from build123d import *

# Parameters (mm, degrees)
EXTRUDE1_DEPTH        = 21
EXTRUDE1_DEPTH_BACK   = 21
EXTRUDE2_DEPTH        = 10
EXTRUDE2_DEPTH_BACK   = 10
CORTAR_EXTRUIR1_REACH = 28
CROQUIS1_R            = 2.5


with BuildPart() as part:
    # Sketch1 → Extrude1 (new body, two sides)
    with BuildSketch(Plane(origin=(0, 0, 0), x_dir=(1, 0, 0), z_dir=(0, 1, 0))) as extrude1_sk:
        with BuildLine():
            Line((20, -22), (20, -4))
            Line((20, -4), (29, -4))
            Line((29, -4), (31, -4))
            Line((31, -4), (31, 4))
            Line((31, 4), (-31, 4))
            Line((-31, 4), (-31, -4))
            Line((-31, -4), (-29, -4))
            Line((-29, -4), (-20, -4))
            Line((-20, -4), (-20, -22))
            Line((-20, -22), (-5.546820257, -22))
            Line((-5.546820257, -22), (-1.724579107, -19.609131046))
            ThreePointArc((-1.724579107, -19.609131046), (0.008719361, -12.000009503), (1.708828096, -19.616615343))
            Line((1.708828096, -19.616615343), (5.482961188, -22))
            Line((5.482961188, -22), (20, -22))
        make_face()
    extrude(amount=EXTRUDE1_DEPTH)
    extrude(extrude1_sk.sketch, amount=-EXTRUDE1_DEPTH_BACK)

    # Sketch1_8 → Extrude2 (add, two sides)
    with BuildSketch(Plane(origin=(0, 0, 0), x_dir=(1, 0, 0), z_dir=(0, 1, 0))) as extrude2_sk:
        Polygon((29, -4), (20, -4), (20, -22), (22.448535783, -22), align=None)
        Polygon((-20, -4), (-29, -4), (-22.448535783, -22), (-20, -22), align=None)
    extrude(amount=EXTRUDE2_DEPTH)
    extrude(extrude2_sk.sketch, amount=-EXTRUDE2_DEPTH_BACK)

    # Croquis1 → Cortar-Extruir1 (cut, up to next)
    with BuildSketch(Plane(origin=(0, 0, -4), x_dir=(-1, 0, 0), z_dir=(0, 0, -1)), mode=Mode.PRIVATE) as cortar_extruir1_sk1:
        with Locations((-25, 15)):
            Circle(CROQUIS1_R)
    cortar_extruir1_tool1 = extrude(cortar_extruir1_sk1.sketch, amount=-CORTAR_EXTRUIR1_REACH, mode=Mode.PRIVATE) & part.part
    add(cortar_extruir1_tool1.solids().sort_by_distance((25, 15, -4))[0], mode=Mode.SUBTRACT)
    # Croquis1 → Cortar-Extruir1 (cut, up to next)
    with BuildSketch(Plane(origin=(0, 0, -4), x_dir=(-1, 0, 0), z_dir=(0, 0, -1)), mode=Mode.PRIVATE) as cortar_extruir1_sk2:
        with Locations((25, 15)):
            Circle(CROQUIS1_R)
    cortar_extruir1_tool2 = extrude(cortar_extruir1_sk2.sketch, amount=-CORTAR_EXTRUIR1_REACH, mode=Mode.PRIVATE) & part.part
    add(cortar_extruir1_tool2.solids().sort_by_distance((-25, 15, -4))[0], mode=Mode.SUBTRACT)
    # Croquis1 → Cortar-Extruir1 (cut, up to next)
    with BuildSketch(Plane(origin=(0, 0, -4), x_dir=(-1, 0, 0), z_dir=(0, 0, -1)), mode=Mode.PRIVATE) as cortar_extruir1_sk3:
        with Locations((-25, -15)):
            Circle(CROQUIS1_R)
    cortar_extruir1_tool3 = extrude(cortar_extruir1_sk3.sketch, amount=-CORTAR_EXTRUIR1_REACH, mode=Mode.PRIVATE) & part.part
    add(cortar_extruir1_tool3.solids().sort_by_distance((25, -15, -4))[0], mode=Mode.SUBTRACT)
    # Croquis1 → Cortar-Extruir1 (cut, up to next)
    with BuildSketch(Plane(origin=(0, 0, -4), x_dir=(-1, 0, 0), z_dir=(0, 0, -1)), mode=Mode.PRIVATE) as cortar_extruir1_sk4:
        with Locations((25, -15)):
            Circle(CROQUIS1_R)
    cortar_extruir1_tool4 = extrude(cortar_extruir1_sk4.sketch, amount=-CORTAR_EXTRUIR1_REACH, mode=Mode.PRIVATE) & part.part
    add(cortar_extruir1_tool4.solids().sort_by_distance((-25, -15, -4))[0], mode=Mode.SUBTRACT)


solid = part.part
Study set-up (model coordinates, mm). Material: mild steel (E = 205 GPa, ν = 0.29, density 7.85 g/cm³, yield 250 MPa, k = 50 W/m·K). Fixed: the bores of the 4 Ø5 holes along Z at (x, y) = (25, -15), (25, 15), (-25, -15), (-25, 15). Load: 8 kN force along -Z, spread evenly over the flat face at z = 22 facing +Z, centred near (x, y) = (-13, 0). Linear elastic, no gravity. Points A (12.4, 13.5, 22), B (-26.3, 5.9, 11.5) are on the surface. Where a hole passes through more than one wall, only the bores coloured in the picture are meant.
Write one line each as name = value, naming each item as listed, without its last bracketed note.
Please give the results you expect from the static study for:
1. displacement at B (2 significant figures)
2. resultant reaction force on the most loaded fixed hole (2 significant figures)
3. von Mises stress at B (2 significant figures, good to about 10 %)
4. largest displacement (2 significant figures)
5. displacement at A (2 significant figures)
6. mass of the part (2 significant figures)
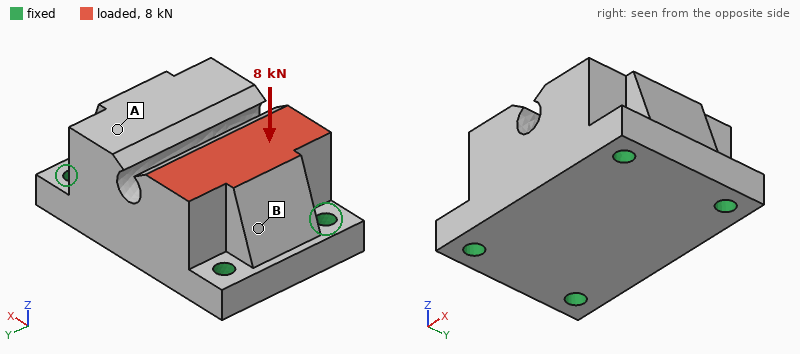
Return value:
displacement at B = 2.3 µm
resultant reaction force on the most loaded fixed hole = 3.3 kN
von Mises stress at B = 14 MPa
largest displacement = 4.0 µm
displacement at A = 2.5 µm
mass of the part = 410 g
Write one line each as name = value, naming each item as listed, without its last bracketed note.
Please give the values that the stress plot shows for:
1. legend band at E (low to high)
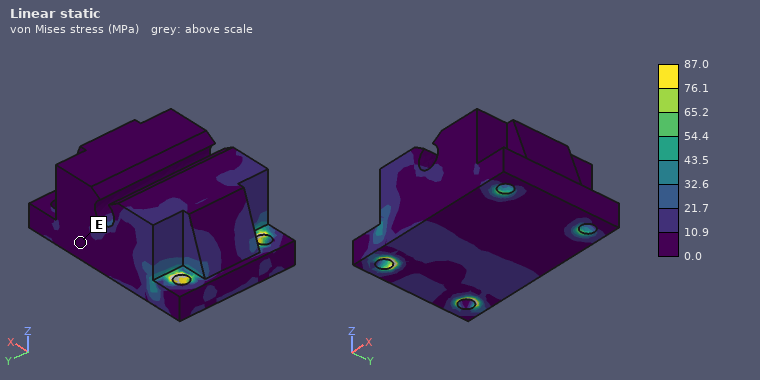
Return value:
legend band at E = 0.0 to 10.9 MPa
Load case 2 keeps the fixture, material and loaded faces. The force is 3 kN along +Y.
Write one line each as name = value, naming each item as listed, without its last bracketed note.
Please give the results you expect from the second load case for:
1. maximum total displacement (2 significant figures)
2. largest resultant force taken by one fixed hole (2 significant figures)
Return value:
maximum total displacement = 4.7 µm
largest resultant force taken by one fixed hole = 1.8 kN
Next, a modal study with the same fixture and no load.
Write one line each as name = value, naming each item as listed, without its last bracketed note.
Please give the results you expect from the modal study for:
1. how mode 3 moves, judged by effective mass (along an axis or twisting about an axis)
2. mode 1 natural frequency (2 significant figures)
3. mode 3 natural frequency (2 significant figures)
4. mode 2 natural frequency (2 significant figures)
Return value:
how mode 3 moves, judged by effective mass = along X
mode 1 natural frequency = 13 kHz
mode 3 natural frequency = 20 kHz
mode 2 natural frequency = 14 kHz
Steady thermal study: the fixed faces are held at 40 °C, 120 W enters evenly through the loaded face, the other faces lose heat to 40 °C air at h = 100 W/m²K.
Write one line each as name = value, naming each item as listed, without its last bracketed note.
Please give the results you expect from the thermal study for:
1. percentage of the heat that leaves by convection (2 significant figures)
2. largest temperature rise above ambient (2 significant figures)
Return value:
percentage of the heat that leaves by convection = 22 %
largest temperature rise above ambient = 85 K
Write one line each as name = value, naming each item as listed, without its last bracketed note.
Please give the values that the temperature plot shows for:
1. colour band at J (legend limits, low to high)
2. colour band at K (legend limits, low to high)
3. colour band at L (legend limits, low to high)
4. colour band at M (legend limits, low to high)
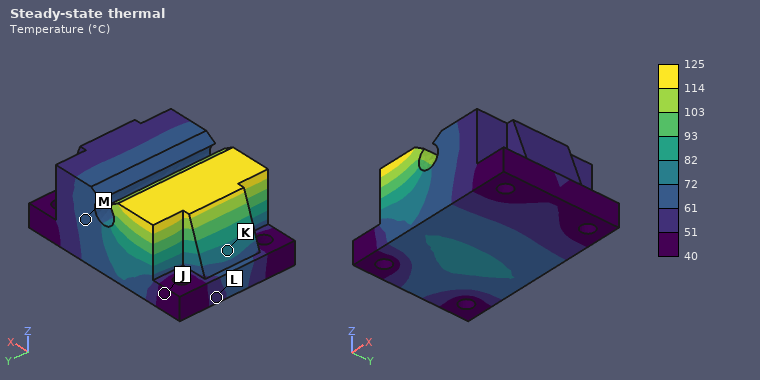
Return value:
colour band at J = 40 to 51 °C
colour band at K = 72 to 82 °C
colour band at L = 51 to 61 °C
colour band at M = 61 to 72 °C
